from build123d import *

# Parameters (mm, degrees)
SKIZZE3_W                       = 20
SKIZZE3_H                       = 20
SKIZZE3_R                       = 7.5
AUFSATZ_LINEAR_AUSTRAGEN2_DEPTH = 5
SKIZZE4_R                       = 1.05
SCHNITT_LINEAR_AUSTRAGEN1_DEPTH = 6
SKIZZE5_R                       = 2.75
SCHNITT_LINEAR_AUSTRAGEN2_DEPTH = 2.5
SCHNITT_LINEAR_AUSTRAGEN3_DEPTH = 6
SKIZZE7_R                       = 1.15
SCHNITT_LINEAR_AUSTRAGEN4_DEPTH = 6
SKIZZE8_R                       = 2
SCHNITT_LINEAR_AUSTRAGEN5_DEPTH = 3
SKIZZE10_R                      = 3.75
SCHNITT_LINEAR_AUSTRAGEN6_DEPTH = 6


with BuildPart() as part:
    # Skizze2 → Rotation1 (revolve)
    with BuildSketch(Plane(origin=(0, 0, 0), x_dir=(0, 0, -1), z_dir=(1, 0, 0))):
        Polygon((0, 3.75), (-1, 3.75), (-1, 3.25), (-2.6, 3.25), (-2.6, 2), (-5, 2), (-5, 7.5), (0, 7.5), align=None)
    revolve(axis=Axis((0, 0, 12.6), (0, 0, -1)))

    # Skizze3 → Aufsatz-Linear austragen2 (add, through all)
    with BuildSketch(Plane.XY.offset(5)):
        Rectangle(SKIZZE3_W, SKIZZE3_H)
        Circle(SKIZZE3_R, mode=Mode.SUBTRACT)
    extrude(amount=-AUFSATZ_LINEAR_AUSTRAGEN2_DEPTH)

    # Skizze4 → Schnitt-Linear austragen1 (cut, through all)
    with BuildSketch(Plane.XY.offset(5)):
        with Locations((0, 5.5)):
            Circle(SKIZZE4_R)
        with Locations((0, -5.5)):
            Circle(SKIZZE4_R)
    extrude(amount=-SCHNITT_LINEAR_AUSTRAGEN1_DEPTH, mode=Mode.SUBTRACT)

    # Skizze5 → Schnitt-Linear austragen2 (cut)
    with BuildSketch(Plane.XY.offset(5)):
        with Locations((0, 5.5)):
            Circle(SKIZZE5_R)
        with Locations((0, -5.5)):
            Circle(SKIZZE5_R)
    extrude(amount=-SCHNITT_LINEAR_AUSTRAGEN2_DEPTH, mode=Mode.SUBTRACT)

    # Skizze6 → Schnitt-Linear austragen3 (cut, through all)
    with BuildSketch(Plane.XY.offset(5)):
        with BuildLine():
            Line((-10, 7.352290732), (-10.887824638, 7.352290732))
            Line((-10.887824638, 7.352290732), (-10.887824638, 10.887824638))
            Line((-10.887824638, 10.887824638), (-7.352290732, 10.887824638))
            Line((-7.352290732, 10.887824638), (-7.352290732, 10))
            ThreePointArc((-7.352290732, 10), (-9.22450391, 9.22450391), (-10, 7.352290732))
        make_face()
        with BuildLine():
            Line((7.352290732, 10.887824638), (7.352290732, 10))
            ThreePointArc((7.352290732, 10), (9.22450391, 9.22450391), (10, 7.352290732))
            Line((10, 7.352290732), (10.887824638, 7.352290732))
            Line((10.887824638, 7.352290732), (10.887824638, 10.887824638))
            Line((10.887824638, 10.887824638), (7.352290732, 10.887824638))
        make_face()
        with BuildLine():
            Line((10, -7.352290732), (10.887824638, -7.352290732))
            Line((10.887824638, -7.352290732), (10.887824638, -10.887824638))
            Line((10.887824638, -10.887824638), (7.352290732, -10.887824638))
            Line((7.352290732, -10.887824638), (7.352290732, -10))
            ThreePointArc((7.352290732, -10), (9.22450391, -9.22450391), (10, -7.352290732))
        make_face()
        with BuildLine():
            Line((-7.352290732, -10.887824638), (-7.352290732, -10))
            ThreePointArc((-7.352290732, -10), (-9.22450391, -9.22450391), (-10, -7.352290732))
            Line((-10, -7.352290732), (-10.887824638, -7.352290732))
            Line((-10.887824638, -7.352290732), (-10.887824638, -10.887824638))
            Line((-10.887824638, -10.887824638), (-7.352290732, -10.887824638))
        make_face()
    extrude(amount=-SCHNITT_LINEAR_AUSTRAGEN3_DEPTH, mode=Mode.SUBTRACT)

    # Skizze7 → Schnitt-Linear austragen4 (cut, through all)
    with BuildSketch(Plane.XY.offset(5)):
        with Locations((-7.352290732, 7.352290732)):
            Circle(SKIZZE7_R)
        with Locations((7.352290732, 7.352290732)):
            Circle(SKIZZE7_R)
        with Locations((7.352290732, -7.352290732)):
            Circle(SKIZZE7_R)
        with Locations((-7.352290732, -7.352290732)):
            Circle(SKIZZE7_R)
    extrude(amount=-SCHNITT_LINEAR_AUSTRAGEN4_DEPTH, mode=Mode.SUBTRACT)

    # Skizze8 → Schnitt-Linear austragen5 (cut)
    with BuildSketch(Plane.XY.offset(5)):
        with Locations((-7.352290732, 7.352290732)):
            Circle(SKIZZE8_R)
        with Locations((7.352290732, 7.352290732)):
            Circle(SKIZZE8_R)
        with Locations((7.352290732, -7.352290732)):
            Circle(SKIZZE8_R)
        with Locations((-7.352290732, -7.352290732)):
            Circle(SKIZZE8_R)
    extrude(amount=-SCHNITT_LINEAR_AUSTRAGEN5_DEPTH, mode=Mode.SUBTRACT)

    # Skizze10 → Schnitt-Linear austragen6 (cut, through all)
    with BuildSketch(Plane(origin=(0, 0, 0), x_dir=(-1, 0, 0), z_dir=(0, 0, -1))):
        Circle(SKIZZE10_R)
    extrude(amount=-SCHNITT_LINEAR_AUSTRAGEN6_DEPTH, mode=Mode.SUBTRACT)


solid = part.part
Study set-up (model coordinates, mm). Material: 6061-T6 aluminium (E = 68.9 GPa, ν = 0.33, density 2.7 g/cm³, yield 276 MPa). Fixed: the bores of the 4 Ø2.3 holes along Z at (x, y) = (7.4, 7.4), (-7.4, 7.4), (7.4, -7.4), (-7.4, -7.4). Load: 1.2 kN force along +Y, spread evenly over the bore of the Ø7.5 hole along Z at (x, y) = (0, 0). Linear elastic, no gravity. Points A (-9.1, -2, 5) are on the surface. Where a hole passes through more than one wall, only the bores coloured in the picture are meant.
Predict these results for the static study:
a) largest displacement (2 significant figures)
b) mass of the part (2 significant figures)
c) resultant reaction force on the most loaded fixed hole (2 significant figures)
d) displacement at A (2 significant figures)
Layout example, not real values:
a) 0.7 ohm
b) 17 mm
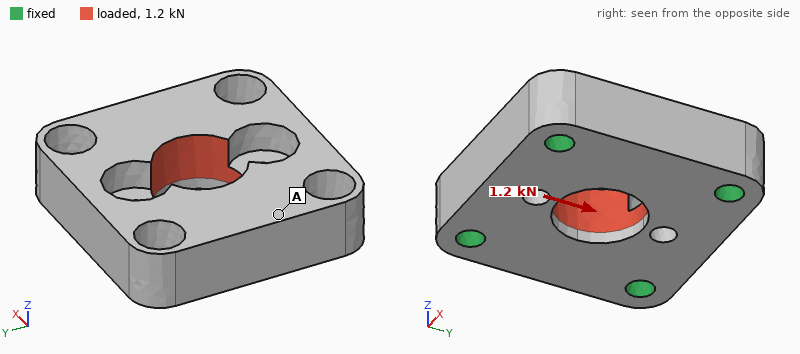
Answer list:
a) 3.7 µm
b) 3.9 g
c) 330 N
d) 0.94 µm
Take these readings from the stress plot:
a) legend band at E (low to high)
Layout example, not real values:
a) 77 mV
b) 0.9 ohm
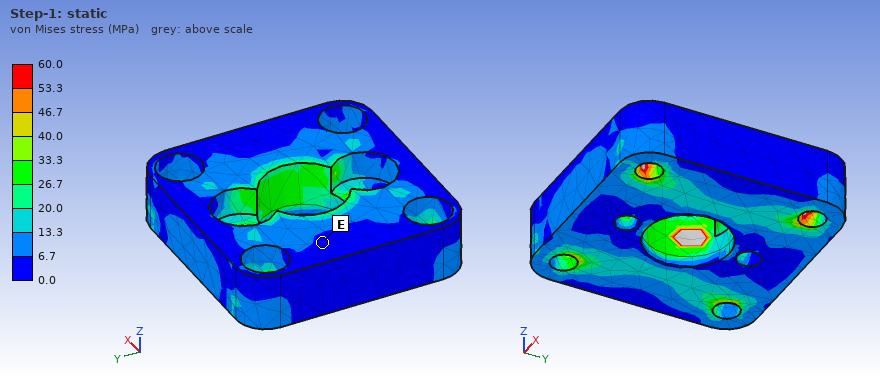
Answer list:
a) 0.0 to 6.7 MPa
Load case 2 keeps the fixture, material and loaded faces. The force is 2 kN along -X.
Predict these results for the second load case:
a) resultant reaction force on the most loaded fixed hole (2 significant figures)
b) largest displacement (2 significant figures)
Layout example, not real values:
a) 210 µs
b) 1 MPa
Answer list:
a) 530 N
b) 8.3 µm
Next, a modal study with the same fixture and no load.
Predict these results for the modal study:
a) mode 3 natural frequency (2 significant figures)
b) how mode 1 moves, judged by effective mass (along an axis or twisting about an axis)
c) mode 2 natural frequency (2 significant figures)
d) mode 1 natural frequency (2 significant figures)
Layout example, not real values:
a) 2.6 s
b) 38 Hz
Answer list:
a) 61 kHz
b) along Z
c) 59 kHz
d) 43 kHz
